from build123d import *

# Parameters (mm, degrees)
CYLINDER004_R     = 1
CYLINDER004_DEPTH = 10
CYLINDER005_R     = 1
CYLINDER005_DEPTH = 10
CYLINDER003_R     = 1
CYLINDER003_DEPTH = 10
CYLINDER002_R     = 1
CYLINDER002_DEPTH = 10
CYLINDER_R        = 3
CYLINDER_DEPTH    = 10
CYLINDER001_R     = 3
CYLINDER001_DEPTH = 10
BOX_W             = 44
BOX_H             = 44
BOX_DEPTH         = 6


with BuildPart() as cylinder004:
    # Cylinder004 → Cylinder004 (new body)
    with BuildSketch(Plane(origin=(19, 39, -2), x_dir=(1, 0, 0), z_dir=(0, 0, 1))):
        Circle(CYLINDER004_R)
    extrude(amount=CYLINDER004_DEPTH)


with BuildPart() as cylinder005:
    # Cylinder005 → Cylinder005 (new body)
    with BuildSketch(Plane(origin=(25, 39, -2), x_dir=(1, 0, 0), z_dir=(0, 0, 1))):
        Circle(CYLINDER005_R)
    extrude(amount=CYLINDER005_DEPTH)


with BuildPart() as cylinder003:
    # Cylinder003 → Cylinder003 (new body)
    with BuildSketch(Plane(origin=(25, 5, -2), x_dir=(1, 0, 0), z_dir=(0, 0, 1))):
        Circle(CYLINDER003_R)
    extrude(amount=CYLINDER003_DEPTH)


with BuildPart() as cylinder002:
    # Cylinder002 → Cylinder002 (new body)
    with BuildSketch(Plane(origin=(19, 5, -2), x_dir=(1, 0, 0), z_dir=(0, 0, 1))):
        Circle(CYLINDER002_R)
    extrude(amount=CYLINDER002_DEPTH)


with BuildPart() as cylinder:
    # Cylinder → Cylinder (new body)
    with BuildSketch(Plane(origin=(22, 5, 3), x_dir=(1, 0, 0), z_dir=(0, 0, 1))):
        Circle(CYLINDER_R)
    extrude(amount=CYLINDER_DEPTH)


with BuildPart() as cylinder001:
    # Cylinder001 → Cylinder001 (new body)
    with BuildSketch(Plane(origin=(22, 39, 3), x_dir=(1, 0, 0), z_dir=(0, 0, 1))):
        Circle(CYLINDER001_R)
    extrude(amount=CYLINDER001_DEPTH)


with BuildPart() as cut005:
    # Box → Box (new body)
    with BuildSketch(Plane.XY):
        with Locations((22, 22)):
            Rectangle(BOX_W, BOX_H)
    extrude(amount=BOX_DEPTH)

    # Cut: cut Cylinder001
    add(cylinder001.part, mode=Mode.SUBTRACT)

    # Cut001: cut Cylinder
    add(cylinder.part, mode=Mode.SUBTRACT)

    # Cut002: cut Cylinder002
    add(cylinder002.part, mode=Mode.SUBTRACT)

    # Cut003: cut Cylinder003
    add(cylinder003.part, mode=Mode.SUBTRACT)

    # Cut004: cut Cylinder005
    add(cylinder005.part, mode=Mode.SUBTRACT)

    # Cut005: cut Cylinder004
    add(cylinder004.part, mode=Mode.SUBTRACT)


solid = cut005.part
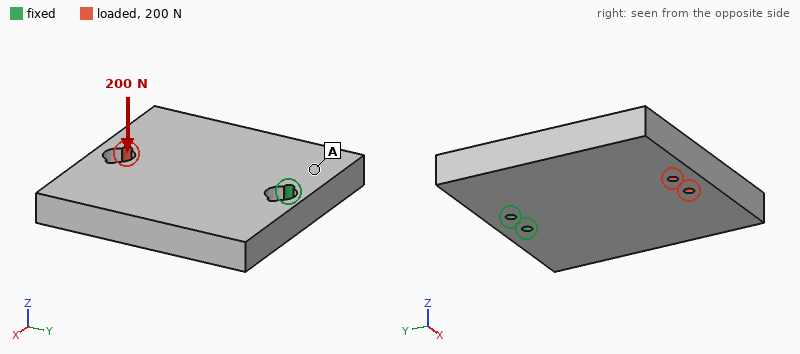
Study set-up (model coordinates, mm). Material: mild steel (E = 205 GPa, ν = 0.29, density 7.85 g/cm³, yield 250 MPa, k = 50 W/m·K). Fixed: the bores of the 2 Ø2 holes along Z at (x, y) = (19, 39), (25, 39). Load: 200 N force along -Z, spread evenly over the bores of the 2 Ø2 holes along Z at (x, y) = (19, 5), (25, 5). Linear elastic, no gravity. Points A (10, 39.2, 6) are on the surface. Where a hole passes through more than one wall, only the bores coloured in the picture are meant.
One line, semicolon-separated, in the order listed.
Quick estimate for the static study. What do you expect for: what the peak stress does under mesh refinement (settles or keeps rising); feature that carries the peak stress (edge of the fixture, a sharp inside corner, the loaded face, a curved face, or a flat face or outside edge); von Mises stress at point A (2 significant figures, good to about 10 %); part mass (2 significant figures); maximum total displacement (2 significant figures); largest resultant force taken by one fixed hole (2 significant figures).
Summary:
keeps rising; edge of the fixture; 15 MPa; 89 g; 35 µm; 100 N
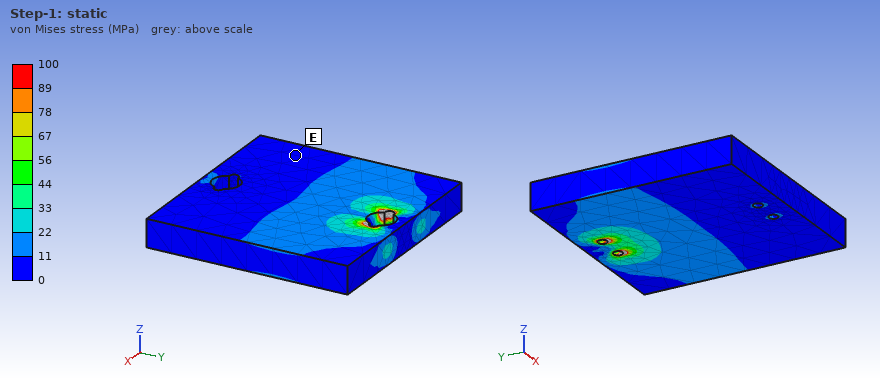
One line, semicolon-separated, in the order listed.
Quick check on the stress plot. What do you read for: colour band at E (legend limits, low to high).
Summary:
0 to 11 MPa
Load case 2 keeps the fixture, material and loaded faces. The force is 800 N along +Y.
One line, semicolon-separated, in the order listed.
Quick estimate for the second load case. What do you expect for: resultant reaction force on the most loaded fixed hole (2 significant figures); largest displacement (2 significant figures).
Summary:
400 N; 2.4 µm
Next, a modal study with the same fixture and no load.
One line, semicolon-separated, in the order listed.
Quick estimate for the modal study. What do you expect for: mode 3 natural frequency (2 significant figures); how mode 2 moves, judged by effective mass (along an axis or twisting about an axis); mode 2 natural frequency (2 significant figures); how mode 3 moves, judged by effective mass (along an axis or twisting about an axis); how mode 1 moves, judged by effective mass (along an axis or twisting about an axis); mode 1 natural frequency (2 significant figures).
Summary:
4400 Hz; along X; 3900 Hz; twisting about Y; along Z; 2400 Hz
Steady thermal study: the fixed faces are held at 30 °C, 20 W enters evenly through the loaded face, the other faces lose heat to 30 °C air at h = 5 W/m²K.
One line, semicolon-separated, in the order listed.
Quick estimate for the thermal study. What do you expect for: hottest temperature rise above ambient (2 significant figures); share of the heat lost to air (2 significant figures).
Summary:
84 K; 4.8 %
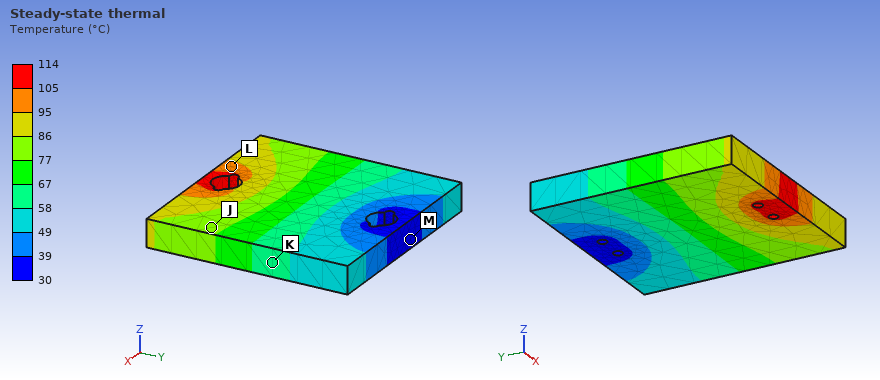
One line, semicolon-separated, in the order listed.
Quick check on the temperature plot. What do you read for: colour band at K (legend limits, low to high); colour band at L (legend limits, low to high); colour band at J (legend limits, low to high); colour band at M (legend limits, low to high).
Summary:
58 to 67 °C; 95 to 105 °C; 77 to 86 °C; 30 to 39 °C
